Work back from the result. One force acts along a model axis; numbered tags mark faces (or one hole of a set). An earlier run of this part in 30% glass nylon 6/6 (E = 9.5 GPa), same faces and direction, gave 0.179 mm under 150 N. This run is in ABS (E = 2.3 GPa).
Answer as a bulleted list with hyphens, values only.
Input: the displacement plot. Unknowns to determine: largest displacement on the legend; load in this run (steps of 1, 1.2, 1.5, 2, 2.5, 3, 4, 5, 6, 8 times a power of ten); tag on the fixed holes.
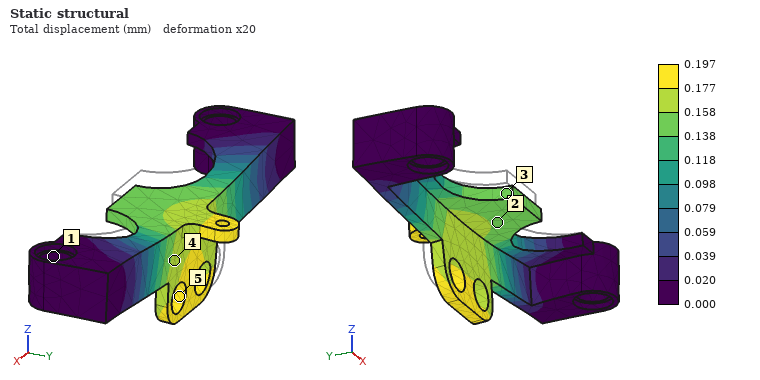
- 0.197 mm
- 40 N
- 1
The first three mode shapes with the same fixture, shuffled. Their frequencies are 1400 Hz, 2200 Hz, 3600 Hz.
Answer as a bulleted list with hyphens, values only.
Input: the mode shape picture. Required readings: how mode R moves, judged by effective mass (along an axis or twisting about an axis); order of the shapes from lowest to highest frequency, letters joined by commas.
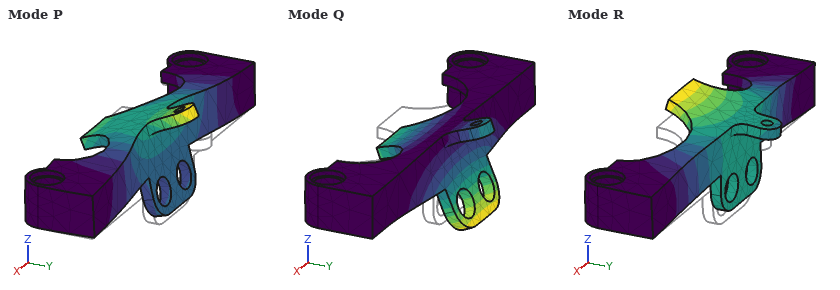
- along Z
- Q, R, P
